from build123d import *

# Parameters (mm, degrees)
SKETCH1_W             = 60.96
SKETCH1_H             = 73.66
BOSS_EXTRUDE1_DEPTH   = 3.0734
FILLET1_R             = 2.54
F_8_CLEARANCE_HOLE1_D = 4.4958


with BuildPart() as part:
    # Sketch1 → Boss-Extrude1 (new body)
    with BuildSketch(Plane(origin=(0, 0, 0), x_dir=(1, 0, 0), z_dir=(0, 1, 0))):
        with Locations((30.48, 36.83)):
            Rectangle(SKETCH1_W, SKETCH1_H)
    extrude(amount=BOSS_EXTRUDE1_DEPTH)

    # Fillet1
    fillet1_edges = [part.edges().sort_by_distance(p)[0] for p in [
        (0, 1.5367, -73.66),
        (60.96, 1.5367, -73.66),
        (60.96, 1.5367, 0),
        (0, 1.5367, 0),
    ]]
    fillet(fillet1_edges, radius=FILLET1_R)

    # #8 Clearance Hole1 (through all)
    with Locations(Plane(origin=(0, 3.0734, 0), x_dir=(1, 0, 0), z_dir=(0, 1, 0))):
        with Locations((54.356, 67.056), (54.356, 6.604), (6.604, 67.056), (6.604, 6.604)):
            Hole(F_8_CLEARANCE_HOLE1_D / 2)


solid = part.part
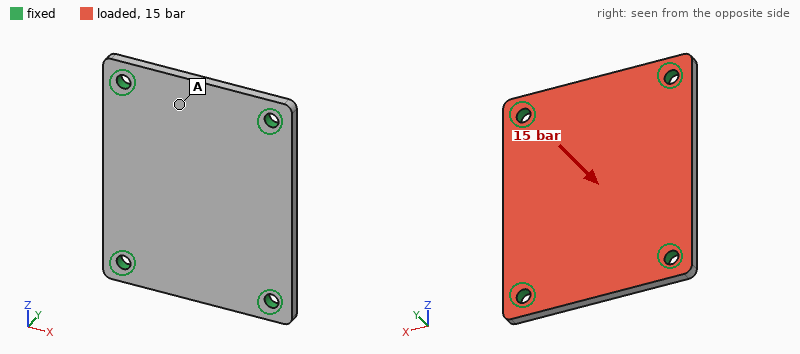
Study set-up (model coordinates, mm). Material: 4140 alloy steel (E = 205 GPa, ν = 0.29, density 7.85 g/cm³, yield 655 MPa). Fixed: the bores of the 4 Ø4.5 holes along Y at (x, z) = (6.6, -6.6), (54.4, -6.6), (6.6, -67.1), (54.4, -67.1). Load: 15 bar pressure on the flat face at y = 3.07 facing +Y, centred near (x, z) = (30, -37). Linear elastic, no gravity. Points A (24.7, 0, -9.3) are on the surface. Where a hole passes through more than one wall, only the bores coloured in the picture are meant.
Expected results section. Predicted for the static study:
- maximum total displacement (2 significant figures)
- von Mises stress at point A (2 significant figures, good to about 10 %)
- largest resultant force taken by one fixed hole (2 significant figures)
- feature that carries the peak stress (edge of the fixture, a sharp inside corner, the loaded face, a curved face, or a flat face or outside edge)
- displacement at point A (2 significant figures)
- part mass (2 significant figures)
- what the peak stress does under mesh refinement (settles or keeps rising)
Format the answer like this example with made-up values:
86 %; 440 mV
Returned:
0.17 mm; 110 MPa; 1.7 kN; edge of the fixture; 0.060 mm; 110 g; keeps rising
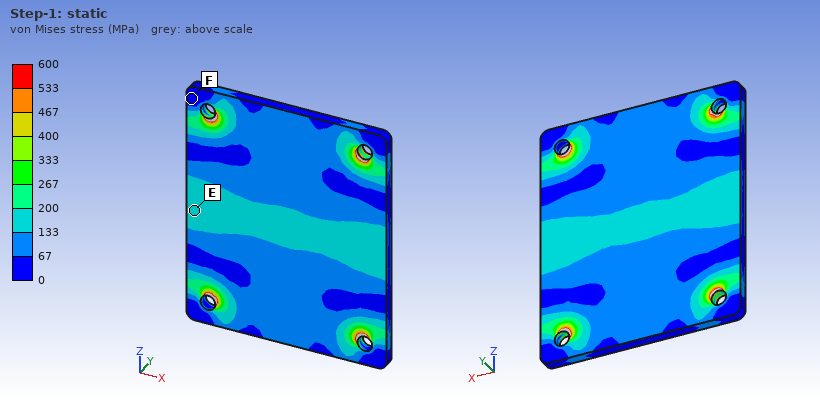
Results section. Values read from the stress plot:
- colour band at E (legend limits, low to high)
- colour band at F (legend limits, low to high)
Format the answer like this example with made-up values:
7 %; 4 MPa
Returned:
133 to 200 MPa; 0 to 67 MPa
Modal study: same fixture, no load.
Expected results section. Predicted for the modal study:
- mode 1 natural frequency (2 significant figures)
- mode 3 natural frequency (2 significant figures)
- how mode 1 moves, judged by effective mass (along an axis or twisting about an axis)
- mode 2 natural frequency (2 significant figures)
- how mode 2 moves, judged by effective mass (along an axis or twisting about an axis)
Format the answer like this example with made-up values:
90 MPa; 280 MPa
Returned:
3700 Hz; 7000 Hz; along Y; 5400 Hz; twisting about Z
